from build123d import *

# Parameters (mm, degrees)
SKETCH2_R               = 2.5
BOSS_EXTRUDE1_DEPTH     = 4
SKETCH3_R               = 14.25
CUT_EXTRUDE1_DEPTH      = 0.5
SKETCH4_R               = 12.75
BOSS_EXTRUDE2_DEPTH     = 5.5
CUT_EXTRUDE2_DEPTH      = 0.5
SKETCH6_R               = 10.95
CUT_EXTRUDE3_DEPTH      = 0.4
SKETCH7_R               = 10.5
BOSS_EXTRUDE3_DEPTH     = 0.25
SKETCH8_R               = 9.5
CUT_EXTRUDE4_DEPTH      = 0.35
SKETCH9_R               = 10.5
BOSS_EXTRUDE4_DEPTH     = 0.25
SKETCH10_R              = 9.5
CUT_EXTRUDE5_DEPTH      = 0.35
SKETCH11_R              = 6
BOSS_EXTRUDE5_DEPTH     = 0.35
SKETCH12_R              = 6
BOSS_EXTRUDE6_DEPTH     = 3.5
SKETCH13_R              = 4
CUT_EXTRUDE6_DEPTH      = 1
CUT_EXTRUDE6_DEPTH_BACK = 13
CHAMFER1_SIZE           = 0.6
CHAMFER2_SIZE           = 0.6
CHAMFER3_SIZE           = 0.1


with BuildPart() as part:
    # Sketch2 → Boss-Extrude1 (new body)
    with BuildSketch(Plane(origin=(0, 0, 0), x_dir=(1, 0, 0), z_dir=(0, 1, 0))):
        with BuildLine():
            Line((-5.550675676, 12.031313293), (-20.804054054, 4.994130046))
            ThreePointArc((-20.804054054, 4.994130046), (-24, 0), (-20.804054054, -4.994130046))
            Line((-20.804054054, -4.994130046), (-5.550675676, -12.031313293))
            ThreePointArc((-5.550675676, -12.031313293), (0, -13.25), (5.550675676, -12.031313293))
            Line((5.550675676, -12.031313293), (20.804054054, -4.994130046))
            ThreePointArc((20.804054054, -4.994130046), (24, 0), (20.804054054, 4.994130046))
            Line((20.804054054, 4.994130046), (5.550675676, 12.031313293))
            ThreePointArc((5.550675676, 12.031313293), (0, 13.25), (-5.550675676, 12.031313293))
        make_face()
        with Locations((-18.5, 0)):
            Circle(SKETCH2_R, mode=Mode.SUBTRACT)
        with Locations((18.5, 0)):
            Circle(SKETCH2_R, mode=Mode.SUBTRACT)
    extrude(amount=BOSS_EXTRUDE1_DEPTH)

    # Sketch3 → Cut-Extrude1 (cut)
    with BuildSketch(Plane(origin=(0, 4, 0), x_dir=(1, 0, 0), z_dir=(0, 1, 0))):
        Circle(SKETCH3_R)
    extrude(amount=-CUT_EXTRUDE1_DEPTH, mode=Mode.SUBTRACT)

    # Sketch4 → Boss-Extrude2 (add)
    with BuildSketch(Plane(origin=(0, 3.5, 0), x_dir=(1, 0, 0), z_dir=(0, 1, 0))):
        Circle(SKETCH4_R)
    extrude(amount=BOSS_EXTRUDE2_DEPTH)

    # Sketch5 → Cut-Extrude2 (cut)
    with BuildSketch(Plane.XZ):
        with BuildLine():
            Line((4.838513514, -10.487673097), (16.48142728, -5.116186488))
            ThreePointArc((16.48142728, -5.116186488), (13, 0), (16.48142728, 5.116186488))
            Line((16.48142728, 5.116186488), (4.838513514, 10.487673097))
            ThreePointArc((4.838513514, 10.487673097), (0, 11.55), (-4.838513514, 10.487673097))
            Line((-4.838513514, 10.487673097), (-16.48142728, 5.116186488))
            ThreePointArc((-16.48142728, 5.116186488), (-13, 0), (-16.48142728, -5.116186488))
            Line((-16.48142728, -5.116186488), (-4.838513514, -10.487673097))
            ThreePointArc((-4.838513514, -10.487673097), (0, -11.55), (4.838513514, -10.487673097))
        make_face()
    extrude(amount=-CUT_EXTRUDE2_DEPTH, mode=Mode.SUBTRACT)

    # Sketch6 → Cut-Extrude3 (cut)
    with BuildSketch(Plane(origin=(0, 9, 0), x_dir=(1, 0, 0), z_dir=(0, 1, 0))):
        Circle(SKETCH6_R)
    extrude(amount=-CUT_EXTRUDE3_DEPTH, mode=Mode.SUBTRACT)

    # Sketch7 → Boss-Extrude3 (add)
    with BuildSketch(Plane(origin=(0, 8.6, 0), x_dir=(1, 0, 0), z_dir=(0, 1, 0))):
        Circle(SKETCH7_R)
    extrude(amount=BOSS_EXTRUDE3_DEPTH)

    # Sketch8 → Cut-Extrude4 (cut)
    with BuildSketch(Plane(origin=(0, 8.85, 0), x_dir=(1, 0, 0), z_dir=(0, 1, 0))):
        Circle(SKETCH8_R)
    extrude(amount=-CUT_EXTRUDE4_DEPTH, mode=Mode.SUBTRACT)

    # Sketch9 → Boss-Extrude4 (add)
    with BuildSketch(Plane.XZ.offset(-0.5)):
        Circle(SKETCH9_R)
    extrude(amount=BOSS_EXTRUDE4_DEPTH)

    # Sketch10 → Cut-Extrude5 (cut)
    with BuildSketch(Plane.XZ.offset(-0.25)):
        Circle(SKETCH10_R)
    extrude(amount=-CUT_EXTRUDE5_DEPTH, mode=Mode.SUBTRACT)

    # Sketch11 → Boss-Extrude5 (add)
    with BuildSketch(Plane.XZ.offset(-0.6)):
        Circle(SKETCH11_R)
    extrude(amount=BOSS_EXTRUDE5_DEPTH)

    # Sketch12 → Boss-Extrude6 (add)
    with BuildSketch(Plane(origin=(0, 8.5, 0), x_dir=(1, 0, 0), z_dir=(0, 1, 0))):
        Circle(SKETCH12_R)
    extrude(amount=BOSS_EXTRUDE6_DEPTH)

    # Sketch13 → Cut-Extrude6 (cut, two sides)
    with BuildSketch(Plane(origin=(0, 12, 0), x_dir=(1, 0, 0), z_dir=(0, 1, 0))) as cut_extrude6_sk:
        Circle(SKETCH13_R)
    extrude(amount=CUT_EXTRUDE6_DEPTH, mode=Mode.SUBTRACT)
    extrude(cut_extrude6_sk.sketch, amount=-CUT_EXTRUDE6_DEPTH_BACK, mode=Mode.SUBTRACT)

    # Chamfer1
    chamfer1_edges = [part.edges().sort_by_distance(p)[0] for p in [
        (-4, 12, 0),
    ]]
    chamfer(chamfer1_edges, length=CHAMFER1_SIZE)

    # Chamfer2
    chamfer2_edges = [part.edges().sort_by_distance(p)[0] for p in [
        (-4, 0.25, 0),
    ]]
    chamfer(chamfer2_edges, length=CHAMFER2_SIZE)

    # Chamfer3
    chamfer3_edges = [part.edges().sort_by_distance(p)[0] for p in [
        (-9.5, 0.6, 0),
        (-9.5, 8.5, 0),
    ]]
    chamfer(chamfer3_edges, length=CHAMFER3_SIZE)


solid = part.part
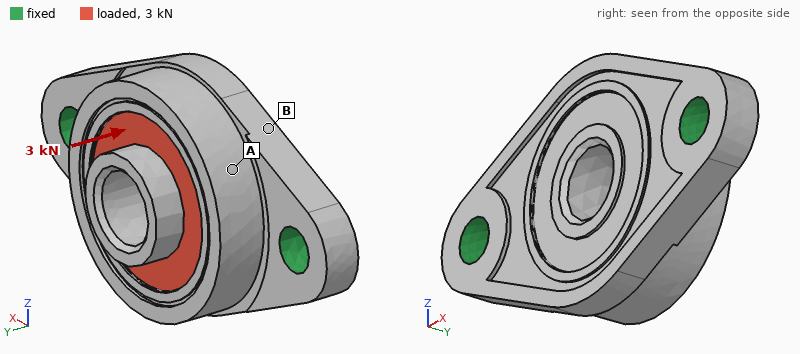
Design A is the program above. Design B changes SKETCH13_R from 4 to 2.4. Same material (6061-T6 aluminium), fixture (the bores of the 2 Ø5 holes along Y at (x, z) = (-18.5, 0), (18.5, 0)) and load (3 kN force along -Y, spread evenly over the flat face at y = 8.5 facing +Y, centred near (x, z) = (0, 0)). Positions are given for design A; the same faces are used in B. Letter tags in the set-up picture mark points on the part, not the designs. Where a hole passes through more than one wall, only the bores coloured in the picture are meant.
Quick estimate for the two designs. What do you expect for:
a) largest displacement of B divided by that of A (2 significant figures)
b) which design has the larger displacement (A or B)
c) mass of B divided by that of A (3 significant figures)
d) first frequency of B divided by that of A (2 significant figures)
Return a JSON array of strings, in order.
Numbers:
["0.90", "A", "1.07", "0.98"]
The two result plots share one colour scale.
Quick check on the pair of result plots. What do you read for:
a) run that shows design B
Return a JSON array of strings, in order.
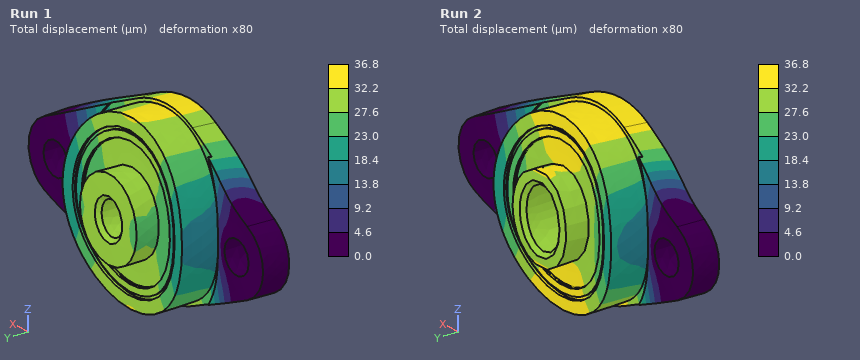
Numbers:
["Run 1"]
